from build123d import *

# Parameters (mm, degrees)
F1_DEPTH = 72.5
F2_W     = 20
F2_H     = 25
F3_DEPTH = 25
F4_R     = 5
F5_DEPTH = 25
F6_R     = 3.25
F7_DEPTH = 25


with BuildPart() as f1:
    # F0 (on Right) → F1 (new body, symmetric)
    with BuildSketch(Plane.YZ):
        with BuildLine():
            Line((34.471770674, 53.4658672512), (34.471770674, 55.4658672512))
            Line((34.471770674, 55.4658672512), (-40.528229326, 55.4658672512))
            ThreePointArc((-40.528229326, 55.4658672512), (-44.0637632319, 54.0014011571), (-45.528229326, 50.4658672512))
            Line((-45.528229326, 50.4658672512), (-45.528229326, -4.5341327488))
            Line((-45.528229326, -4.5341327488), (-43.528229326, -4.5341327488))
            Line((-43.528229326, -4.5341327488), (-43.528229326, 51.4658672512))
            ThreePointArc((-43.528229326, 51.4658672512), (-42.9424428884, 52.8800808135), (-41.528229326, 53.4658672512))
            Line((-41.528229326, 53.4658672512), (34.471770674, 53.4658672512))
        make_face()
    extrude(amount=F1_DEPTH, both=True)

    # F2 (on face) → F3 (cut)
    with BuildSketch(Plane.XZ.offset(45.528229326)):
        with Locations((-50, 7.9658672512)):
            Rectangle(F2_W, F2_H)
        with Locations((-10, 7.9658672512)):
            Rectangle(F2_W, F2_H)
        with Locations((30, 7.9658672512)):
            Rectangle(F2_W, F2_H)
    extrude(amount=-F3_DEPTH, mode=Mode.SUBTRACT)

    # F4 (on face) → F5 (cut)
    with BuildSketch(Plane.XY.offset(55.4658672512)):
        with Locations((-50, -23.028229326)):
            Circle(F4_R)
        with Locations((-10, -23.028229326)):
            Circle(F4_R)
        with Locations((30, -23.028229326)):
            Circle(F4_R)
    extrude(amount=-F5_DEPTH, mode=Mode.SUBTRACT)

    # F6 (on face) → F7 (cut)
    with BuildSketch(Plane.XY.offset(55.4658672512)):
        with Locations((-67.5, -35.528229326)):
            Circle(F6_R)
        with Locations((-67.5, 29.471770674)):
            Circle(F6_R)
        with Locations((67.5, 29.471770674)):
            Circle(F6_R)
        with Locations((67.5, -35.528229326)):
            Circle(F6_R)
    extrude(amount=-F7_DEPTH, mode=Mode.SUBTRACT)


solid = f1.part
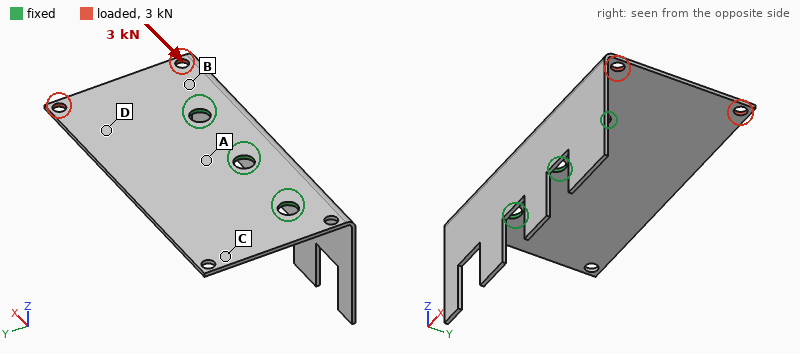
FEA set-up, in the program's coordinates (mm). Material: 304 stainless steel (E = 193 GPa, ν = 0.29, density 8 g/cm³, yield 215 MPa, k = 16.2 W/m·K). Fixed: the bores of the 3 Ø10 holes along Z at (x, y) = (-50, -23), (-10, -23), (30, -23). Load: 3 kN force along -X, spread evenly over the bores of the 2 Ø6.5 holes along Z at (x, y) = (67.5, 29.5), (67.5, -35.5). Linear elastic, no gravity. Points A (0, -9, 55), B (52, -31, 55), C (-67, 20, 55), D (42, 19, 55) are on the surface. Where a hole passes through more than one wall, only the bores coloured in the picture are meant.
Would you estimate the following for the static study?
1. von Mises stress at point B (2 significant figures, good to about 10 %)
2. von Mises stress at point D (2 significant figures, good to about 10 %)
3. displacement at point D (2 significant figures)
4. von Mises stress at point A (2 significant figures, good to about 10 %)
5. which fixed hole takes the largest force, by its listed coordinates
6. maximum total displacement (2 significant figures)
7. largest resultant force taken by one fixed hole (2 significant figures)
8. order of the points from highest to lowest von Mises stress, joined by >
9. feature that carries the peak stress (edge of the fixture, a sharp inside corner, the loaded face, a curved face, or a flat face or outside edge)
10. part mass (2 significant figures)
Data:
35 MPa
25 MPa
9.0 µm
18 MPa
(30, -23)
27 µm
1.9 kN
B > D > A > C
the loaded face
290 g
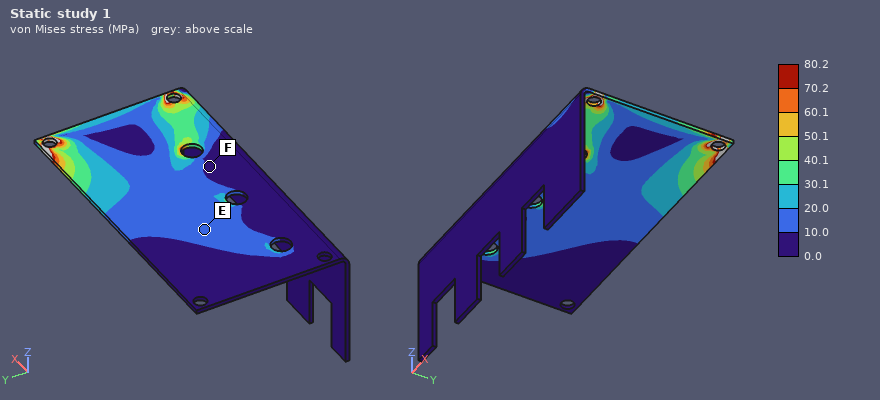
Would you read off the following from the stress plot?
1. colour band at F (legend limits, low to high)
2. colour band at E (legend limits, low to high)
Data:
0.0 to 10.0 MPa
10.0 to 20.0 MPa
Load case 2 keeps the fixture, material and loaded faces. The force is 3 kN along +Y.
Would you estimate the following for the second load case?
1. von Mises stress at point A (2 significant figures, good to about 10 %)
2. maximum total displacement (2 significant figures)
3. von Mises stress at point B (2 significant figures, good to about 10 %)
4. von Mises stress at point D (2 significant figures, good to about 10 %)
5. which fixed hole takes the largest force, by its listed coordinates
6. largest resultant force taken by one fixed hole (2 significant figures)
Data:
19 MPa
44 µm
37 MPa
23 MPa
(30, -23)
4.3 kN
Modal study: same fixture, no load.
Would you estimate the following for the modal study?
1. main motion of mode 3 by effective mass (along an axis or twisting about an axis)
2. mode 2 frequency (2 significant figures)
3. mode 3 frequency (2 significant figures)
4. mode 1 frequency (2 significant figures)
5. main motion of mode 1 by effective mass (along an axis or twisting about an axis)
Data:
along Z
450 Hz
510 Hz
350 Hz
along Y
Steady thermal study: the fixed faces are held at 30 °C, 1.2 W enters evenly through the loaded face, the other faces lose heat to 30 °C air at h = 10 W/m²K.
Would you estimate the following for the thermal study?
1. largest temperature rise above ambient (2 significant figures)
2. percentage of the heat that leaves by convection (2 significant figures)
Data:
28 K
65 %
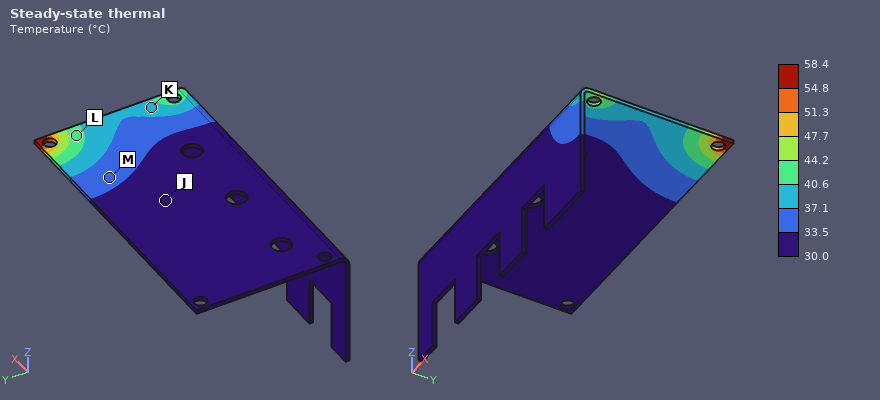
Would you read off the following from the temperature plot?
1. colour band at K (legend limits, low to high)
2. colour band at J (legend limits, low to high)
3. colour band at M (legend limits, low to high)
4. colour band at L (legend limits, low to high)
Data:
37.1 to 40.6 °C
30.0 to 33.5 °C
33.5 to 37.1 °C
40.6 to 44.2 °C
